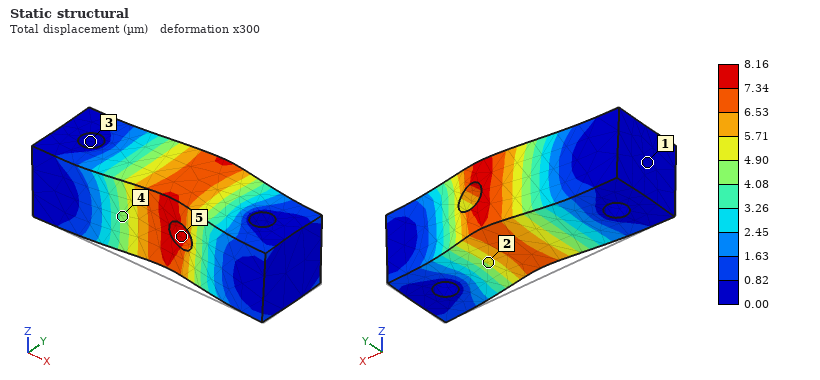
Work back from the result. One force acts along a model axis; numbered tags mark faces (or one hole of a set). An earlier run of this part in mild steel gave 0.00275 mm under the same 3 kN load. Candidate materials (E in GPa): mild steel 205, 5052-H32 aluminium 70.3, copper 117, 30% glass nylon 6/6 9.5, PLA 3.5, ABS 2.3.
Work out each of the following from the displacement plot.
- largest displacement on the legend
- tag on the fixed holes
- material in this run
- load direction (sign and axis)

8.16 µm
3
5052-H32 aluminium
+Z
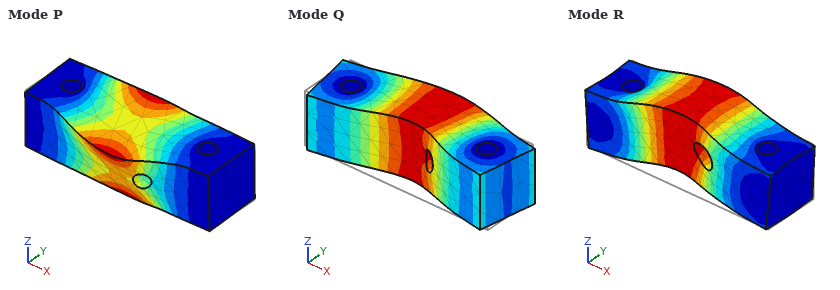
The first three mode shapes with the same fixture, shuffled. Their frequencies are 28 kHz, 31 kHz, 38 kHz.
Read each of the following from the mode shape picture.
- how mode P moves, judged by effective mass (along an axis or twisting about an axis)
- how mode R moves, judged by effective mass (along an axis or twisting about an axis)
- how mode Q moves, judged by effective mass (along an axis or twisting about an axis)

twisting about X
along Z
along Y
